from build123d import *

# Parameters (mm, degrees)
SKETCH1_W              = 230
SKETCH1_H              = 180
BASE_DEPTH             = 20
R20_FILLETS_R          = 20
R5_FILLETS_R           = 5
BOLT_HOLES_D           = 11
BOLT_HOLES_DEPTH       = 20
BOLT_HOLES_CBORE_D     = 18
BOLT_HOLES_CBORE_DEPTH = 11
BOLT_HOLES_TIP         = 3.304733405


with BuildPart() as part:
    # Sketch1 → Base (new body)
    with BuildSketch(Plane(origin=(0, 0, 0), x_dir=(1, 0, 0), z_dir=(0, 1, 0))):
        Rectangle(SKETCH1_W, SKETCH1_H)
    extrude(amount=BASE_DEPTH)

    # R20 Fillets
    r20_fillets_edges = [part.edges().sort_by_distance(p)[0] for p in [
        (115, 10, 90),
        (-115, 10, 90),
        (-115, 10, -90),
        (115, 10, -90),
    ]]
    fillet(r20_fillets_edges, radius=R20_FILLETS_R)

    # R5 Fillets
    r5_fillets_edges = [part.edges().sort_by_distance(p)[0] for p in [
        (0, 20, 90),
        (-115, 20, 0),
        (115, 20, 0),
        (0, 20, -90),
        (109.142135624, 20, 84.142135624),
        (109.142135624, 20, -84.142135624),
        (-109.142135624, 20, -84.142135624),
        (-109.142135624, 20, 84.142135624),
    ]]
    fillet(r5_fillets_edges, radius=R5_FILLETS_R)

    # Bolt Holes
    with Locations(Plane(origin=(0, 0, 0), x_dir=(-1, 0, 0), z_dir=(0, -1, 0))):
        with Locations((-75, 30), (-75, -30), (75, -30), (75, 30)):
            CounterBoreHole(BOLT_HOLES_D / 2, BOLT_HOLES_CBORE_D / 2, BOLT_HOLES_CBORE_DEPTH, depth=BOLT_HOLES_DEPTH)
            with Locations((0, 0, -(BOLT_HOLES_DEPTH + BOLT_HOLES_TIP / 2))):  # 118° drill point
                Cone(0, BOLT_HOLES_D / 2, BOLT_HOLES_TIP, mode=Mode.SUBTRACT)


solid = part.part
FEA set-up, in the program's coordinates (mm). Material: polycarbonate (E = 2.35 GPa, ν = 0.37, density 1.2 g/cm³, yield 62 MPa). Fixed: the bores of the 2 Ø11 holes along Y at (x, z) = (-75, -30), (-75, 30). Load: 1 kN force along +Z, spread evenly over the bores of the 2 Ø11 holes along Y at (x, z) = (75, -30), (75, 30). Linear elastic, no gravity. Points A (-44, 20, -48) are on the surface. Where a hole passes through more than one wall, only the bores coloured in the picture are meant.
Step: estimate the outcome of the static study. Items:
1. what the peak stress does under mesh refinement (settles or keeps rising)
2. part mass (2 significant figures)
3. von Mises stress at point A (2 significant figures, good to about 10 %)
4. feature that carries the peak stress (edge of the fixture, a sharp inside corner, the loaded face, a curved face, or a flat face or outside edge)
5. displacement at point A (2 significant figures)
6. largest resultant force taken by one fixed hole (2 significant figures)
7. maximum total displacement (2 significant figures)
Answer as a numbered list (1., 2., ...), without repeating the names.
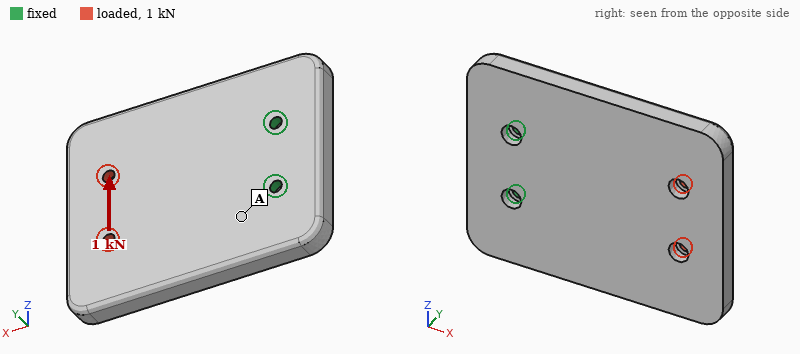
1. keeps rising
2. 960 g
3. 1.5 MPa
4. edge of the fixture
5. 0.13 mm
6. 2.3 kN
7. 0.59 mm
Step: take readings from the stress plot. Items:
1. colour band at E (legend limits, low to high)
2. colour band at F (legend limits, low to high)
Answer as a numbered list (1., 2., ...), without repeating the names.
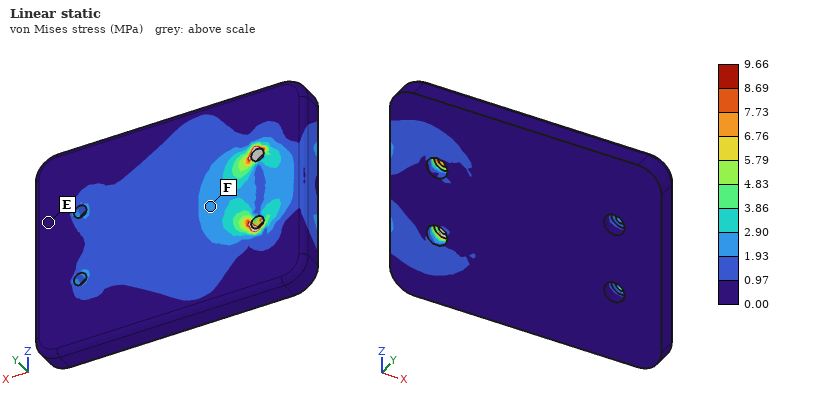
1. 0.00 to 0.97 MPa
2. 1.93 to 2.90 MPa
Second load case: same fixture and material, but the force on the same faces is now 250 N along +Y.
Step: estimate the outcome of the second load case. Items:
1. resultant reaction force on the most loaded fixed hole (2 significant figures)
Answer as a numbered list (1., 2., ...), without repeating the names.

1. 170 N
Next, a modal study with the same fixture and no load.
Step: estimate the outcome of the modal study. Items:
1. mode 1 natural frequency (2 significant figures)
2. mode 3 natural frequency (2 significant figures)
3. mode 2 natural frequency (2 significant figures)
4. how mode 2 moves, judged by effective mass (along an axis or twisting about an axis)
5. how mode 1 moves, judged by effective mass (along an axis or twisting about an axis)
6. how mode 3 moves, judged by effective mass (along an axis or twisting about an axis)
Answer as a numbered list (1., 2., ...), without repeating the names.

1. 83 Hz
2. 370 Hz
3. 250 Hz
4. twisting about X
5. along Y
6. along Z
